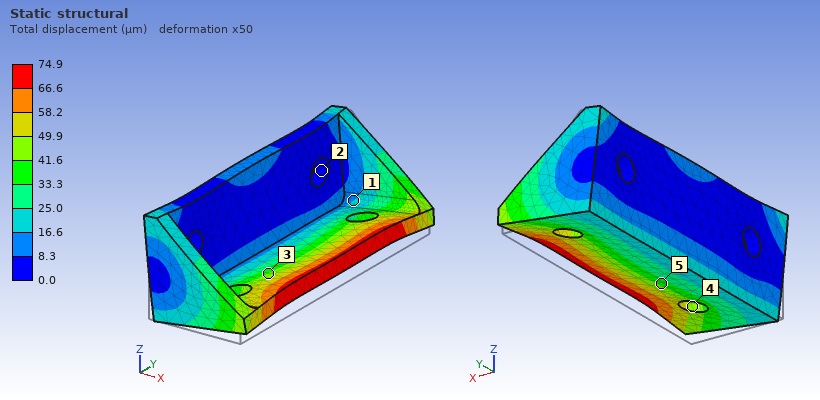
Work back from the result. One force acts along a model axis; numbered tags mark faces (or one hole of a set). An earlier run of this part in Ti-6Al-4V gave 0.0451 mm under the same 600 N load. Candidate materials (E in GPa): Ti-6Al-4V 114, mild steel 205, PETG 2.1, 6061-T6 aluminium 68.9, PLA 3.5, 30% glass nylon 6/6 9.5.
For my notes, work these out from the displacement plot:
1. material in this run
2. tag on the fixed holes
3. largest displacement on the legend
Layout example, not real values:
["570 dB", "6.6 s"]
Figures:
["6061-T6 aluminium", "2", "74.9 µm"]
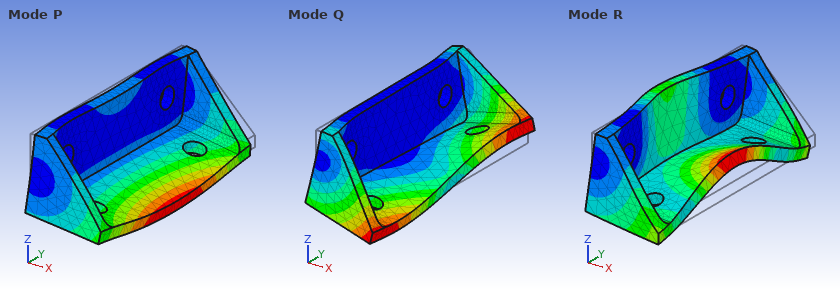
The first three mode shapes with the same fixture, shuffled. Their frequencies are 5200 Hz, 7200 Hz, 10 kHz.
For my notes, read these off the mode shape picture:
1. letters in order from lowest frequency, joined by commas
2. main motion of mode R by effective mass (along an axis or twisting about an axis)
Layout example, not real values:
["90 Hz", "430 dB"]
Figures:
["P, Q, R", "along X"]
